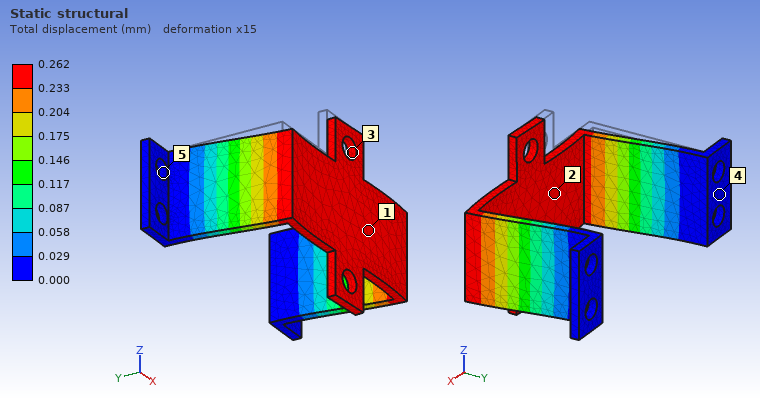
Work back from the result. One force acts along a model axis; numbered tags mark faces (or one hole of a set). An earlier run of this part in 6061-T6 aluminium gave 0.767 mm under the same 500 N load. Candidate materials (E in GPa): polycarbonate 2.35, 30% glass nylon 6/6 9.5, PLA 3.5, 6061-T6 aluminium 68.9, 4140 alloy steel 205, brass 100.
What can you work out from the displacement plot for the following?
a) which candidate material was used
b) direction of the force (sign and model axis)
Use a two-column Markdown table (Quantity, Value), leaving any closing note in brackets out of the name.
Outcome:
| Quantity | Value |
|---|---|
| which candidate material was used | 4140 alloy steel |
| direction of the force | +X |
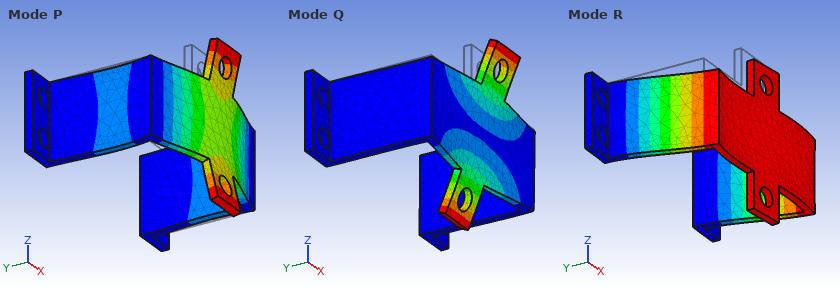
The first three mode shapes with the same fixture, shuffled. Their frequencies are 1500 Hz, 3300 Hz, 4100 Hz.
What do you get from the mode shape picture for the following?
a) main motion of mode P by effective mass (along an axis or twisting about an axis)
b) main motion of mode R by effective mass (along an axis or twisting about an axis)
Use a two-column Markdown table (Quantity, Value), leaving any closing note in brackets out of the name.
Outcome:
| Quantity | Value |
|---|---|
| main motion of mode P by effective mass | along Y |
| main motion of mode R by effective mass | along X |
